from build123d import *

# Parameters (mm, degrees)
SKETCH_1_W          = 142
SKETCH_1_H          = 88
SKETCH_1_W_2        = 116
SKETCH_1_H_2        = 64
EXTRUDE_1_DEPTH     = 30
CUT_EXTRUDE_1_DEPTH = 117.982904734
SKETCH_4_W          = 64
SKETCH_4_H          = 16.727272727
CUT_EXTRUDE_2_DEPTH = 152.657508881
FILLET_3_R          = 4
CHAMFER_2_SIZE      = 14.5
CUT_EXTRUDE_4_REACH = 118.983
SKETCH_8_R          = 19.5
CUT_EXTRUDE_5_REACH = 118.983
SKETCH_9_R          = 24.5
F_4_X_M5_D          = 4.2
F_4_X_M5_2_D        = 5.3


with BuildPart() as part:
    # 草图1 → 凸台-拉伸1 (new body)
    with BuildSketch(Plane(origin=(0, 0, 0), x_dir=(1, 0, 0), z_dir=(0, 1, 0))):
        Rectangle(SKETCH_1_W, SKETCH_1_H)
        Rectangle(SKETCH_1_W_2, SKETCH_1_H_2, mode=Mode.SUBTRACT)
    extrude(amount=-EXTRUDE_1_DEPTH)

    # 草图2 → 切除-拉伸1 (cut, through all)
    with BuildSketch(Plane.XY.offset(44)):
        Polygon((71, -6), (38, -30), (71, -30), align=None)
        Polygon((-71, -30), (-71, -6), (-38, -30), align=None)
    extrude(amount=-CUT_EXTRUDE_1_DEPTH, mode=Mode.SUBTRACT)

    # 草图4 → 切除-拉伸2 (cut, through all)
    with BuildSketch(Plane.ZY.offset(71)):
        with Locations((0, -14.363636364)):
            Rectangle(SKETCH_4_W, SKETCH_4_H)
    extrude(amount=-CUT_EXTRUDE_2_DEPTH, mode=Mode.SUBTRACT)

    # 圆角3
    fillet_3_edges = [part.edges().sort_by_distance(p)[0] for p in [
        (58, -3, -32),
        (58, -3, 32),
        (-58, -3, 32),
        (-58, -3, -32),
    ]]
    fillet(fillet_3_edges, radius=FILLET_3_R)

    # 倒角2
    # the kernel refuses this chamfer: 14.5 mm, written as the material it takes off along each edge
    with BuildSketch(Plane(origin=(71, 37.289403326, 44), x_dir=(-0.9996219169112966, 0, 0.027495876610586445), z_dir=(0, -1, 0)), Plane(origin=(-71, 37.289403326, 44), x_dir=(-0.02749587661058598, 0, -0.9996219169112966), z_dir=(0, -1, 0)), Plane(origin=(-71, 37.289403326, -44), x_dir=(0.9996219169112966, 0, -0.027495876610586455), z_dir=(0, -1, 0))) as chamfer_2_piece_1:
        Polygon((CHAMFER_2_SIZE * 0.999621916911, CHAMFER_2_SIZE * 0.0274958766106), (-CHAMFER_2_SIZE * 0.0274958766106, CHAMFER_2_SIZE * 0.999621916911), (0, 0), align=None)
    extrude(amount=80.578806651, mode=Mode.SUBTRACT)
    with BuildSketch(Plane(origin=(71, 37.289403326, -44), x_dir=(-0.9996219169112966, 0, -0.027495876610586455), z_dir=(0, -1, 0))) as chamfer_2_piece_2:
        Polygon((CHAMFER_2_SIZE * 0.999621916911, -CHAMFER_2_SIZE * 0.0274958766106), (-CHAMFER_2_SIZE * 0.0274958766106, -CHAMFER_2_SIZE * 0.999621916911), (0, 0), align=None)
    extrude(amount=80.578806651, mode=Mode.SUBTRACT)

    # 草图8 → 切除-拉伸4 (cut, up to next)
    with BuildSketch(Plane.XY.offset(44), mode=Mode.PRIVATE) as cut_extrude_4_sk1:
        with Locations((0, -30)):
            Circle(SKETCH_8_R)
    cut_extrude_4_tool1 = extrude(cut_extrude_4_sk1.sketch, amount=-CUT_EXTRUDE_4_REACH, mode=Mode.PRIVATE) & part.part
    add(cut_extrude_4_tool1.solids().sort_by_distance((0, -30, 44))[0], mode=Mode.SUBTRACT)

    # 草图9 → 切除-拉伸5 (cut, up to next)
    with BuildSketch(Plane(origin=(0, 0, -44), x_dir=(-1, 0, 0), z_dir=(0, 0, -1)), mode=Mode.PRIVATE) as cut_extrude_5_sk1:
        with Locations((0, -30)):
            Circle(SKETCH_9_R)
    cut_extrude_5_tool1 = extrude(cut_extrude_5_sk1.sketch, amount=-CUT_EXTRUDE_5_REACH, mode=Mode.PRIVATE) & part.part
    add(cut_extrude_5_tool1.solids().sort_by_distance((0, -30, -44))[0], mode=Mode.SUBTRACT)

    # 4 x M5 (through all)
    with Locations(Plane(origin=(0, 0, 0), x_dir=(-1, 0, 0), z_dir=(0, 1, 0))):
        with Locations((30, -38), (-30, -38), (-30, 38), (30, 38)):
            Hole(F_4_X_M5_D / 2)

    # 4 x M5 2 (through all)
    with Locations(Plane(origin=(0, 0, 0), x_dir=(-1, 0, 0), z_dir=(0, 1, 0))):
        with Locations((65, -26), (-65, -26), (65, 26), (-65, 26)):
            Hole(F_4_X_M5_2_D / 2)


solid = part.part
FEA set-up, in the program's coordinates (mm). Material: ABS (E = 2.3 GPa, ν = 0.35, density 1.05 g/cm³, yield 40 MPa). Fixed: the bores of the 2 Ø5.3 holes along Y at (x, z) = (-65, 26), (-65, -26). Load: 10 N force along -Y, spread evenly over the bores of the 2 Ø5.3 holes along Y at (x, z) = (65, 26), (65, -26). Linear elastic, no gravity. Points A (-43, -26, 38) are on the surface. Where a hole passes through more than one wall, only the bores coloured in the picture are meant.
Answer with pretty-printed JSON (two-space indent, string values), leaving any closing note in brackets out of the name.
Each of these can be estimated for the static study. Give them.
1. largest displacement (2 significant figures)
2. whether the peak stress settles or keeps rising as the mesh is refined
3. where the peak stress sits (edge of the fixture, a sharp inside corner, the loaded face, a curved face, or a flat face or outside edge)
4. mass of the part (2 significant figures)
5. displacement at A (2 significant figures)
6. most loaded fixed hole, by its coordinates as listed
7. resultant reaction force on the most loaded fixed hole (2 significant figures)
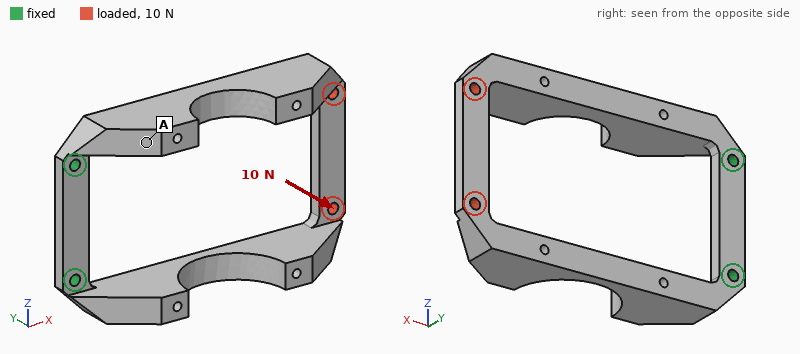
{
  "largest displacement": "2.0 mm",
  "whether the peak stress settles or keeps rising as the mesh is refined": "keeps rising",
  "where the peak stress sits": "a sharp inside corner",
  "mass of the part": "72 g",
  "displacement at A": "0.33 mm",
  "most loaded fixed hole, by its coordinates as listed": "(-65, 26)",
  "resultant reaction force on the most loaded fixed hole": "5.8 N"
}
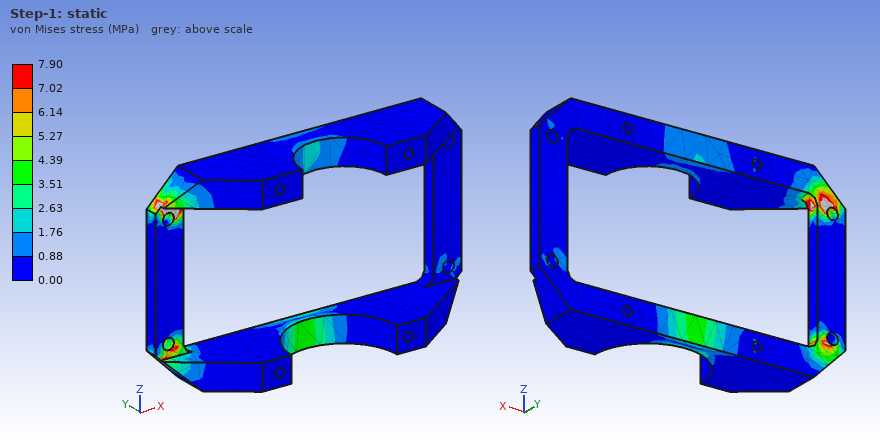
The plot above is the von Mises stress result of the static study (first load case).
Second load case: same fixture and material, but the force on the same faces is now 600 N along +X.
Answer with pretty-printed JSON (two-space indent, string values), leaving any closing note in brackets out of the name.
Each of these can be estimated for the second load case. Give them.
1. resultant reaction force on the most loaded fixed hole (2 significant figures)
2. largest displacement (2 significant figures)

{
  "resultant reaction force on the most loaded fixed hole": "300 N",
  "largest displacement": "1.8 mm"
}
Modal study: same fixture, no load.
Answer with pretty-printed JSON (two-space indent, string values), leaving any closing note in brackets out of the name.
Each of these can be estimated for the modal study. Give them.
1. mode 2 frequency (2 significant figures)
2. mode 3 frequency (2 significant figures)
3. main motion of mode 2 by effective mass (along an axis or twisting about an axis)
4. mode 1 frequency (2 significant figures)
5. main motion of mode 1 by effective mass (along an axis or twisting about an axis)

{
  "mode 2 frequency": "120 Hz",
  "mode 3 frequency": "170 Hz",
  "main motion of mode 2 by effective mass": "along Z",
  "mode 1 frequency": "79 Hz",
  "main motion of mode 1 by effective mass": "along Y"
}
